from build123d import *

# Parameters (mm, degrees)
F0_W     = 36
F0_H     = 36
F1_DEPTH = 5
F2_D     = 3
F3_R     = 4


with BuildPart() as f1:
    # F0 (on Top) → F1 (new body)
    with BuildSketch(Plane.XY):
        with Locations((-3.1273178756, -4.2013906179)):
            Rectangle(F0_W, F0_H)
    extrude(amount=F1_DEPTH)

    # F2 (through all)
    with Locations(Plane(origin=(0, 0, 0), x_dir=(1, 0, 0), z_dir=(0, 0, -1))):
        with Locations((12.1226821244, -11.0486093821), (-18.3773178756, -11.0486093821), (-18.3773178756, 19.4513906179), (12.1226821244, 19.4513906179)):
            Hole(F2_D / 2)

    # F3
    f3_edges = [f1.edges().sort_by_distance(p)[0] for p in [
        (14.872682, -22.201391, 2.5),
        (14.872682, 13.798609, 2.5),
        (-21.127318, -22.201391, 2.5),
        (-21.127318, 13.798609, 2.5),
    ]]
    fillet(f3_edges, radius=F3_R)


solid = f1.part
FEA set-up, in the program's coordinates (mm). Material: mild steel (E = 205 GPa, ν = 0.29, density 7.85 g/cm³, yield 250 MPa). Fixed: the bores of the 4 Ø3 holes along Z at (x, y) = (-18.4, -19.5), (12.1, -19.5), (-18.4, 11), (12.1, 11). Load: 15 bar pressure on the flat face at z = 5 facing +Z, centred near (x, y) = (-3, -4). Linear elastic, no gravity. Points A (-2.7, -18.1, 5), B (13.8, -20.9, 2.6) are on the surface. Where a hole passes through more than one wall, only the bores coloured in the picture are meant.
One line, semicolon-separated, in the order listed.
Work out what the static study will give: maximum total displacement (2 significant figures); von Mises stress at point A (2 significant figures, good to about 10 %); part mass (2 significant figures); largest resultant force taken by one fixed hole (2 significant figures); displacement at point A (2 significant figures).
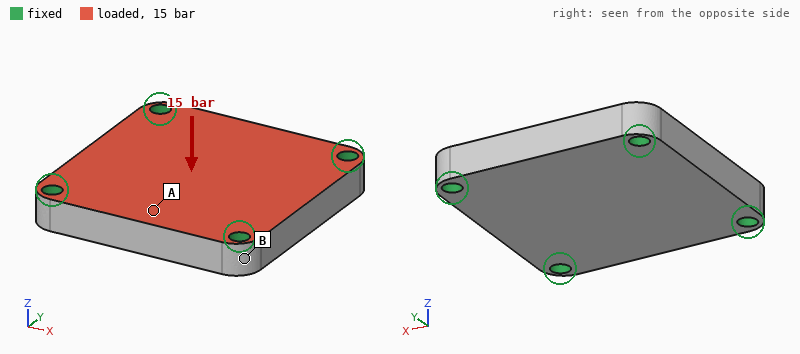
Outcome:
5.0 µm; 17 MPa; 49 g; 470 N; 3.1 µm
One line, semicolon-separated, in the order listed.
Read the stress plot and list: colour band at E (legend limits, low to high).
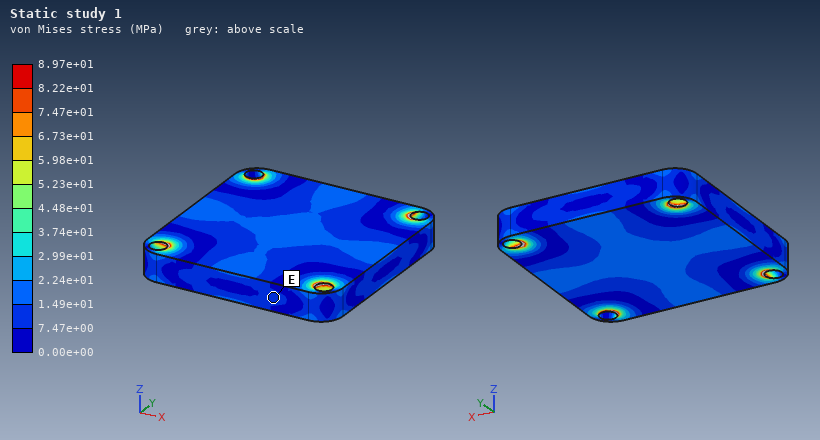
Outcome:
7.47e+00 to 1.49e+01 MPa
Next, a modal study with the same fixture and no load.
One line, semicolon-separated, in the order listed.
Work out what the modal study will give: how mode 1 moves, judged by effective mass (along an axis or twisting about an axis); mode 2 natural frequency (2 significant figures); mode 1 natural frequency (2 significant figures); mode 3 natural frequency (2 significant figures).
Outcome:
along Z; 27 kHz; 17 kHz; 27 kHz
